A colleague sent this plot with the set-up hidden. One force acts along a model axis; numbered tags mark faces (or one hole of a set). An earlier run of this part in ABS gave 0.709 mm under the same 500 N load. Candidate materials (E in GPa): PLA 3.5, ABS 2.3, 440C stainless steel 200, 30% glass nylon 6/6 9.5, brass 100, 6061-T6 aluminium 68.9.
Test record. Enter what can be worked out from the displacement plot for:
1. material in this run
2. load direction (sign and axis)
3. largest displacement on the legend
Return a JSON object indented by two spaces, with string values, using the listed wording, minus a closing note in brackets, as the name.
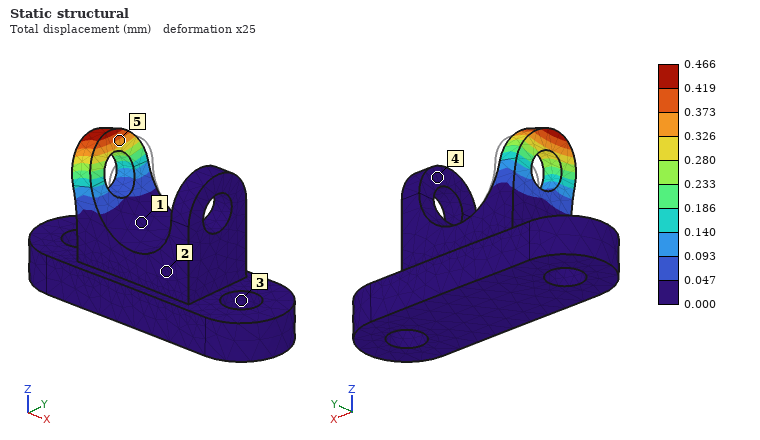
{
  "material in this run": "PLA",
  "load direction": "-X",
  "largest displacement on the legend": "0.466 mm"
}
